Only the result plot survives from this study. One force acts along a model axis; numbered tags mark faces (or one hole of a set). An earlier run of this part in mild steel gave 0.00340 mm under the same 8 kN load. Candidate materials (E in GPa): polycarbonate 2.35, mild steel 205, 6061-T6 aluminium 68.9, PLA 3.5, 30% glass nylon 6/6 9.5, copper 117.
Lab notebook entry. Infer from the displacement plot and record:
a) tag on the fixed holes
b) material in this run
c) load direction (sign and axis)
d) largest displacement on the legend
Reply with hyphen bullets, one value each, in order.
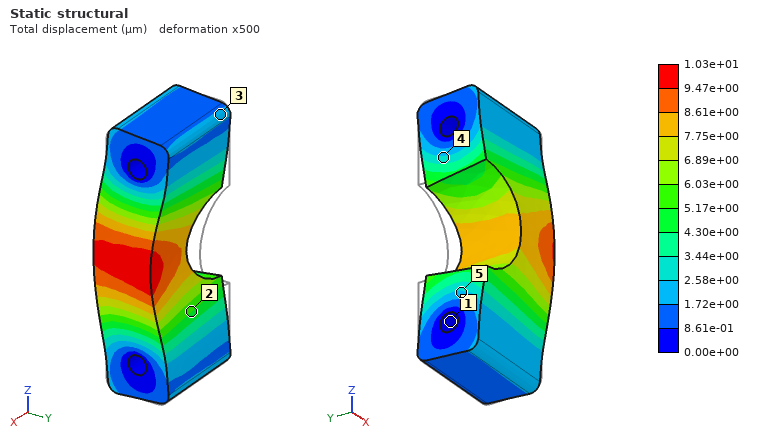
- 1
- 6061-T6 aluminium
- -Y
- 1.03e+01 µm
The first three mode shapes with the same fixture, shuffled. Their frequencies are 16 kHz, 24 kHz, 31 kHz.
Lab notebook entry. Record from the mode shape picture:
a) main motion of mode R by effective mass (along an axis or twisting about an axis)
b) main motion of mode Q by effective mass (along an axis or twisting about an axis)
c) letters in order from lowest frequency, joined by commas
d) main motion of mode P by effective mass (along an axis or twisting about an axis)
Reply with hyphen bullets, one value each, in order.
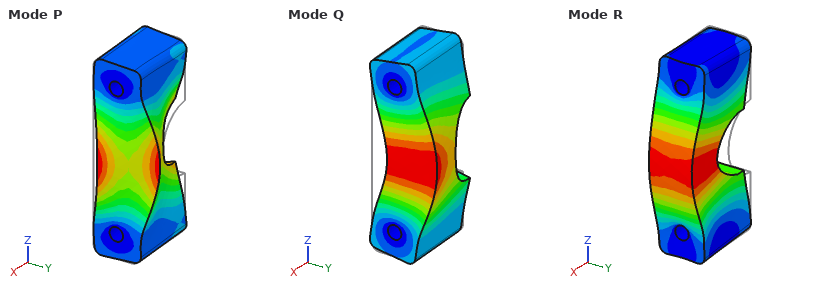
- along X
- along Y
- Q, R, P
- twisting about Z
